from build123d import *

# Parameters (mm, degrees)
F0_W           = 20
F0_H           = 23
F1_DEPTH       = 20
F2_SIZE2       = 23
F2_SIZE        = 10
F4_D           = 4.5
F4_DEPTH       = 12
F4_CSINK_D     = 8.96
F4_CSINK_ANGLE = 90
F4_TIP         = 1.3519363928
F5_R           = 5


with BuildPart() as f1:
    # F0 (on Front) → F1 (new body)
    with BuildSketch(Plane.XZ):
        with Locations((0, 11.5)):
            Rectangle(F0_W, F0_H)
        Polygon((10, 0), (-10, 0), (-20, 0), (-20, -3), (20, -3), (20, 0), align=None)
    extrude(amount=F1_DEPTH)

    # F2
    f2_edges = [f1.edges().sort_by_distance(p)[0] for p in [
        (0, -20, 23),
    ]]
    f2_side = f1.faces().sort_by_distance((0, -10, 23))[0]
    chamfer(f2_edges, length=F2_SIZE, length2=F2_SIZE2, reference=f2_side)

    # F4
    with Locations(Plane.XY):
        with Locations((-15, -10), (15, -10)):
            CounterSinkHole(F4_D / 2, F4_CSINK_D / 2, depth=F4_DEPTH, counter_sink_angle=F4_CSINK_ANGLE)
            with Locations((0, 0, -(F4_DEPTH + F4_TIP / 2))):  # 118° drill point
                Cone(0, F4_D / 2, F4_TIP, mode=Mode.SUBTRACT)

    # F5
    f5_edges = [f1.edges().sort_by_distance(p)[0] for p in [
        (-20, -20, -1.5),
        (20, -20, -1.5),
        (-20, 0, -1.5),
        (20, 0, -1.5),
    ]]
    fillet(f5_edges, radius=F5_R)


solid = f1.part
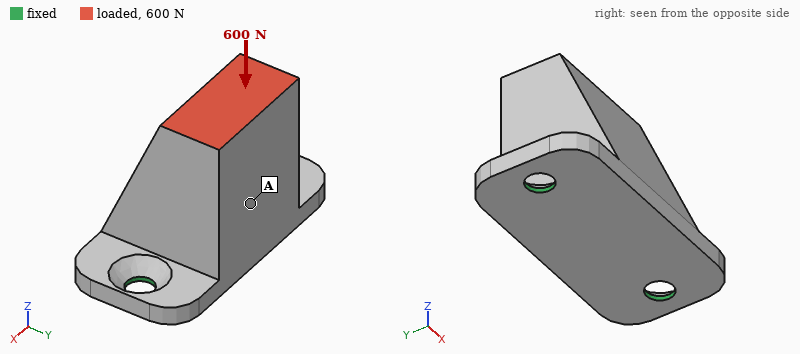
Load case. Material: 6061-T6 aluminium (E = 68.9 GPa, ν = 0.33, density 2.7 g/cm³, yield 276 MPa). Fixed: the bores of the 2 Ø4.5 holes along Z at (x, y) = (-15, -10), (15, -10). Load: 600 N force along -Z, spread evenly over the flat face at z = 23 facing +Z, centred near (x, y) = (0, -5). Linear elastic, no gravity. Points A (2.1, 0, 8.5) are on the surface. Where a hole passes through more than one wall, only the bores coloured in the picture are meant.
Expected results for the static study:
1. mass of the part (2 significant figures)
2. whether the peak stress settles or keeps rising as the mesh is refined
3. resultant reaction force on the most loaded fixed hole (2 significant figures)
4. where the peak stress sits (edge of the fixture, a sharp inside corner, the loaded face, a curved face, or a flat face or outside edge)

24 g
keeps rising
410 N
edge of the fixture
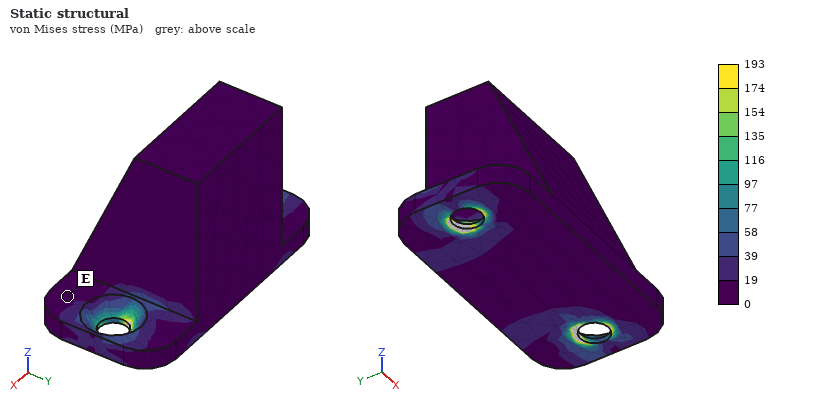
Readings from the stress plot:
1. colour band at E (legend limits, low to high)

0 to 19 MPa
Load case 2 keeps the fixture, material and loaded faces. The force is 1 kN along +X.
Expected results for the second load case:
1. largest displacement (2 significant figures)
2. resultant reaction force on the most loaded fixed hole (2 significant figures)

53 µm
1.1 kN
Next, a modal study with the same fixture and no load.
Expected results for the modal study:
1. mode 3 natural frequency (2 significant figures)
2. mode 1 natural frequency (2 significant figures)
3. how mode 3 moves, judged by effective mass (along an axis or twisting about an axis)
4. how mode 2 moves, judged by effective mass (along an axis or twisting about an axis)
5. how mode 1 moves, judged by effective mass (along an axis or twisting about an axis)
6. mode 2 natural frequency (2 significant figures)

10 kHz
2000 Hz
along Z
along X
along Y
9200 Hz
